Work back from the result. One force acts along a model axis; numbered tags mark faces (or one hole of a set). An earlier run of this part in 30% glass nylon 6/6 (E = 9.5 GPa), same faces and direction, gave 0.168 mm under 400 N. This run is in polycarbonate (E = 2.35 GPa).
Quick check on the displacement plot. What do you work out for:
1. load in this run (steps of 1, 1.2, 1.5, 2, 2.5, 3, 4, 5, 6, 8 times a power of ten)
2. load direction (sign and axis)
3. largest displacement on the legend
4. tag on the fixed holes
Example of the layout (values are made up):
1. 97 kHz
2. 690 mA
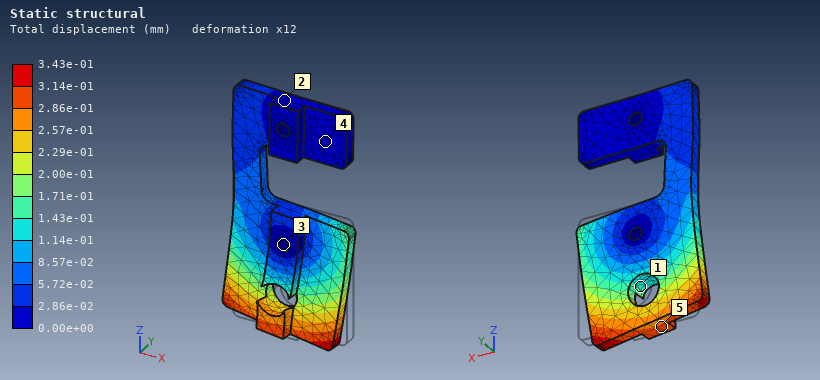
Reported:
1. 200 N
2. -X
3. 3.43e-01 mm
4. 3
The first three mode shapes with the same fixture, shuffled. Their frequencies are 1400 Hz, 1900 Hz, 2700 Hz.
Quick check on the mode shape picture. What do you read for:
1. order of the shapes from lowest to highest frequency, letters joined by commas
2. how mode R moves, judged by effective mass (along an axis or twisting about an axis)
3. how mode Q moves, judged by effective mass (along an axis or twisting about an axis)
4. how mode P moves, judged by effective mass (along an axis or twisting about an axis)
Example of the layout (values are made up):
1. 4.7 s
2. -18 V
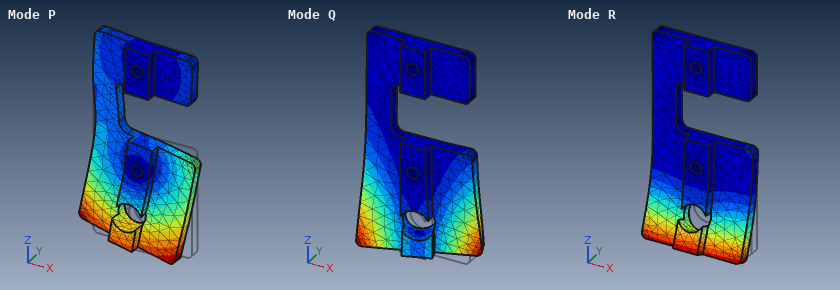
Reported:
1. R, Q, P
2. along Y
3. twisting about Z
4. along X
